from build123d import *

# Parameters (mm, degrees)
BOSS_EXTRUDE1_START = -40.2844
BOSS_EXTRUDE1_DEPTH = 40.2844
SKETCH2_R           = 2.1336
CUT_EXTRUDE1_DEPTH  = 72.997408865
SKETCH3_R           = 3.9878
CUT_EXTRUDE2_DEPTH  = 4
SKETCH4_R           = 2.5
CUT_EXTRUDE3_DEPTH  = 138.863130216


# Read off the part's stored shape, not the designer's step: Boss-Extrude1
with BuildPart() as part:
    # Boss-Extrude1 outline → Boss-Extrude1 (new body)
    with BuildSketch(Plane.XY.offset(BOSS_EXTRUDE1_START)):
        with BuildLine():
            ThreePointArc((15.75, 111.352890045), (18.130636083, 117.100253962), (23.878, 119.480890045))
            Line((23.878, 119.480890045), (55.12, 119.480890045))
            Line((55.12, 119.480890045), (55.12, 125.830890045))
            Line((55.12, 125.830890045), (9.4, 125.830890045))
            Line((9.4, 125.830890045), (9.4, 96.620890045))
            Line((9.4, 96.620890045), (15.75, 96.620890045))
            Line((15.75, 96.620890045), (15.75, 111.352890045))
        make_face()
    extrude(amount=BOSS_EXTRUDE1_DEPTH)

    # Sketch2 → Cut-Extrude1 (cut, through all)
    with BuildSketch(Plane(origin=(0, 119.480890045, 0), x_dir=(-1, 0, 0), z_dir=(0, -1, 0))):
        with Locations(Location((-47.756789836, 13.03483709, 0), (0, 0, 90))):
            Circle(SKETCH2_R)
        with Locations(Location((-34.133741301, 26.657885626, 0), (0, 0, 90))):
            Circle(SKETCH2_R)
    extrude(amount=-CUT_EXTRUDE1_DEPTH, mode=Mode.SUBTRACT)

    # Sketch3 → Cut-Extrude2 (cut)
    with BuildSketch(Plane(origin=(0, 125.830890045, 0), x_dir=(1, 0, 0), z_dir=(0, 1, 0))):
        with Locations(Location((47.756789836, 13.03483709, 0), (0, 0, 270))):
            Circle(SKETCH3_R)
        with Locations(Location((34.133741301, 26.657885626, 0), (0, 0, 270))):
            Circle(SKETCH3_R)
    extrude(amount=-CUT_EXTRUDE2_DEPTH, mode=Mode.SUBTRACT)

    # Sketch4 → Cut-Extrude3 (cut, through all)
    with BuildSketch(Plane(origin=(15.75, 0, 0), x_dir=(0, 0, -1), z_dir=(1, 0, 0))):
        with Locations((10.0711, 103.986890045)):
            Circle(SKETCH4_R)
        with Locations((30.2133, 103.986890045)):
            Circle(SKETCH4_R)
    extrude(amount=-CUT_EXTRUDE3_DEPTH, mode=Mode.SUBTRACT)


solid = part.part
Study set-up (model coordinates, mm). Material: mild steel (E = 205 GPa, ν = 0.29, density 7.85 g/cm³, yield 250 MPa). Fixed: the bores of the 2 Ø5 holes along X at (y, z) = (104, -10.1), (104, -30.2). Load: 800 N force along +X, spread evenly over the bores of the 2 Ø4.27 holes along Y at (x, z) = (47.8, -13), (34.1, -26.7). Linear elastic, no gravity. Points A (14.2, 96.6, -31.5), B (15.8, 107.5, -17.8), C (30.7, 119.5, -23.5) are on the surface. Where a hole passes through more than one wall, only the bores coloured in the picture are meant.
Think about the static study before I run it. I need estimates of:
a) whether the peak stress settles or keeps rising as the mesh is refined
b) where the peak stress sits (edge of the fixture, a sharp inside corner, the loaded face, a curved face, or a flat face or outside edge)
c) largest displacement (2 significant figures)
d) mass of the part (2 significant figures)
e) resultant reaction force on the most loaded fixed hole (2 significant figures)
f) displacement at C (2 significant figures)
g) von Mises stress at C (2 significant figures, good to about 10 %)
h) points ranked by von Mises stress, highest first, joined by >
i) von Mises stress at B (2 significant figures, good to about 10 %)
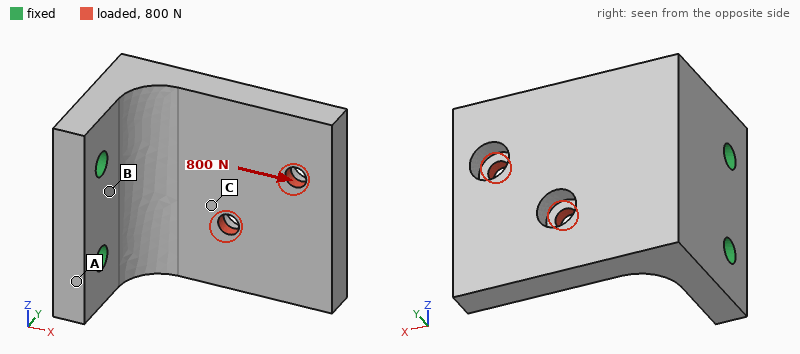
keeps rising
edge of the fixture
23 µm
140 g
410 N
12 µm
12 MPa
B > C > A
24 MPa
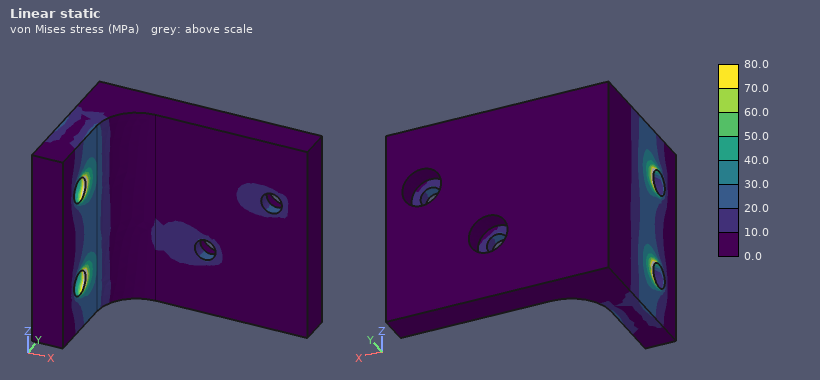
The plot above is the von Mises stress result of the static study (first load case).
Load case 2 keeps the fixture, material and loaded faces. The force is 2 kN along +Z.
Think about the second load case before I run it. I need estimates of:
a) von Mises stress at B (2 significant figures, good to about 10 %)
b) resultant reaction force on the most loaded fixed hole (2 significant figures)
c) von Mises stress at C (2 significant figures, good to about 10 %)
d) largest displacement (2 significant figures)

62 MPa
2.7 kN
47 MPa
73 µm
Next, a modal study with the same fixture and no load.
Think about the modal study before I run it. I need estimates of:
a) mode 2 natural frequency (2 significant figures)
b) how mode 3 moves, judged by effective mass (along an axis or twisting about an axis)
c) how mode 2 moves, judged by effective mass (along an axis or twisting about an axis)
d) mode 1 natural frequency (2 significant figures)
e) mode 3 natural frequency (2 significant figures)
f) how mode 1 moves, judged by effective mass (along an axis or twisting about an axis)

4000 Hz
along X
along Z
2100 Hz
7000 Hz
along Y
